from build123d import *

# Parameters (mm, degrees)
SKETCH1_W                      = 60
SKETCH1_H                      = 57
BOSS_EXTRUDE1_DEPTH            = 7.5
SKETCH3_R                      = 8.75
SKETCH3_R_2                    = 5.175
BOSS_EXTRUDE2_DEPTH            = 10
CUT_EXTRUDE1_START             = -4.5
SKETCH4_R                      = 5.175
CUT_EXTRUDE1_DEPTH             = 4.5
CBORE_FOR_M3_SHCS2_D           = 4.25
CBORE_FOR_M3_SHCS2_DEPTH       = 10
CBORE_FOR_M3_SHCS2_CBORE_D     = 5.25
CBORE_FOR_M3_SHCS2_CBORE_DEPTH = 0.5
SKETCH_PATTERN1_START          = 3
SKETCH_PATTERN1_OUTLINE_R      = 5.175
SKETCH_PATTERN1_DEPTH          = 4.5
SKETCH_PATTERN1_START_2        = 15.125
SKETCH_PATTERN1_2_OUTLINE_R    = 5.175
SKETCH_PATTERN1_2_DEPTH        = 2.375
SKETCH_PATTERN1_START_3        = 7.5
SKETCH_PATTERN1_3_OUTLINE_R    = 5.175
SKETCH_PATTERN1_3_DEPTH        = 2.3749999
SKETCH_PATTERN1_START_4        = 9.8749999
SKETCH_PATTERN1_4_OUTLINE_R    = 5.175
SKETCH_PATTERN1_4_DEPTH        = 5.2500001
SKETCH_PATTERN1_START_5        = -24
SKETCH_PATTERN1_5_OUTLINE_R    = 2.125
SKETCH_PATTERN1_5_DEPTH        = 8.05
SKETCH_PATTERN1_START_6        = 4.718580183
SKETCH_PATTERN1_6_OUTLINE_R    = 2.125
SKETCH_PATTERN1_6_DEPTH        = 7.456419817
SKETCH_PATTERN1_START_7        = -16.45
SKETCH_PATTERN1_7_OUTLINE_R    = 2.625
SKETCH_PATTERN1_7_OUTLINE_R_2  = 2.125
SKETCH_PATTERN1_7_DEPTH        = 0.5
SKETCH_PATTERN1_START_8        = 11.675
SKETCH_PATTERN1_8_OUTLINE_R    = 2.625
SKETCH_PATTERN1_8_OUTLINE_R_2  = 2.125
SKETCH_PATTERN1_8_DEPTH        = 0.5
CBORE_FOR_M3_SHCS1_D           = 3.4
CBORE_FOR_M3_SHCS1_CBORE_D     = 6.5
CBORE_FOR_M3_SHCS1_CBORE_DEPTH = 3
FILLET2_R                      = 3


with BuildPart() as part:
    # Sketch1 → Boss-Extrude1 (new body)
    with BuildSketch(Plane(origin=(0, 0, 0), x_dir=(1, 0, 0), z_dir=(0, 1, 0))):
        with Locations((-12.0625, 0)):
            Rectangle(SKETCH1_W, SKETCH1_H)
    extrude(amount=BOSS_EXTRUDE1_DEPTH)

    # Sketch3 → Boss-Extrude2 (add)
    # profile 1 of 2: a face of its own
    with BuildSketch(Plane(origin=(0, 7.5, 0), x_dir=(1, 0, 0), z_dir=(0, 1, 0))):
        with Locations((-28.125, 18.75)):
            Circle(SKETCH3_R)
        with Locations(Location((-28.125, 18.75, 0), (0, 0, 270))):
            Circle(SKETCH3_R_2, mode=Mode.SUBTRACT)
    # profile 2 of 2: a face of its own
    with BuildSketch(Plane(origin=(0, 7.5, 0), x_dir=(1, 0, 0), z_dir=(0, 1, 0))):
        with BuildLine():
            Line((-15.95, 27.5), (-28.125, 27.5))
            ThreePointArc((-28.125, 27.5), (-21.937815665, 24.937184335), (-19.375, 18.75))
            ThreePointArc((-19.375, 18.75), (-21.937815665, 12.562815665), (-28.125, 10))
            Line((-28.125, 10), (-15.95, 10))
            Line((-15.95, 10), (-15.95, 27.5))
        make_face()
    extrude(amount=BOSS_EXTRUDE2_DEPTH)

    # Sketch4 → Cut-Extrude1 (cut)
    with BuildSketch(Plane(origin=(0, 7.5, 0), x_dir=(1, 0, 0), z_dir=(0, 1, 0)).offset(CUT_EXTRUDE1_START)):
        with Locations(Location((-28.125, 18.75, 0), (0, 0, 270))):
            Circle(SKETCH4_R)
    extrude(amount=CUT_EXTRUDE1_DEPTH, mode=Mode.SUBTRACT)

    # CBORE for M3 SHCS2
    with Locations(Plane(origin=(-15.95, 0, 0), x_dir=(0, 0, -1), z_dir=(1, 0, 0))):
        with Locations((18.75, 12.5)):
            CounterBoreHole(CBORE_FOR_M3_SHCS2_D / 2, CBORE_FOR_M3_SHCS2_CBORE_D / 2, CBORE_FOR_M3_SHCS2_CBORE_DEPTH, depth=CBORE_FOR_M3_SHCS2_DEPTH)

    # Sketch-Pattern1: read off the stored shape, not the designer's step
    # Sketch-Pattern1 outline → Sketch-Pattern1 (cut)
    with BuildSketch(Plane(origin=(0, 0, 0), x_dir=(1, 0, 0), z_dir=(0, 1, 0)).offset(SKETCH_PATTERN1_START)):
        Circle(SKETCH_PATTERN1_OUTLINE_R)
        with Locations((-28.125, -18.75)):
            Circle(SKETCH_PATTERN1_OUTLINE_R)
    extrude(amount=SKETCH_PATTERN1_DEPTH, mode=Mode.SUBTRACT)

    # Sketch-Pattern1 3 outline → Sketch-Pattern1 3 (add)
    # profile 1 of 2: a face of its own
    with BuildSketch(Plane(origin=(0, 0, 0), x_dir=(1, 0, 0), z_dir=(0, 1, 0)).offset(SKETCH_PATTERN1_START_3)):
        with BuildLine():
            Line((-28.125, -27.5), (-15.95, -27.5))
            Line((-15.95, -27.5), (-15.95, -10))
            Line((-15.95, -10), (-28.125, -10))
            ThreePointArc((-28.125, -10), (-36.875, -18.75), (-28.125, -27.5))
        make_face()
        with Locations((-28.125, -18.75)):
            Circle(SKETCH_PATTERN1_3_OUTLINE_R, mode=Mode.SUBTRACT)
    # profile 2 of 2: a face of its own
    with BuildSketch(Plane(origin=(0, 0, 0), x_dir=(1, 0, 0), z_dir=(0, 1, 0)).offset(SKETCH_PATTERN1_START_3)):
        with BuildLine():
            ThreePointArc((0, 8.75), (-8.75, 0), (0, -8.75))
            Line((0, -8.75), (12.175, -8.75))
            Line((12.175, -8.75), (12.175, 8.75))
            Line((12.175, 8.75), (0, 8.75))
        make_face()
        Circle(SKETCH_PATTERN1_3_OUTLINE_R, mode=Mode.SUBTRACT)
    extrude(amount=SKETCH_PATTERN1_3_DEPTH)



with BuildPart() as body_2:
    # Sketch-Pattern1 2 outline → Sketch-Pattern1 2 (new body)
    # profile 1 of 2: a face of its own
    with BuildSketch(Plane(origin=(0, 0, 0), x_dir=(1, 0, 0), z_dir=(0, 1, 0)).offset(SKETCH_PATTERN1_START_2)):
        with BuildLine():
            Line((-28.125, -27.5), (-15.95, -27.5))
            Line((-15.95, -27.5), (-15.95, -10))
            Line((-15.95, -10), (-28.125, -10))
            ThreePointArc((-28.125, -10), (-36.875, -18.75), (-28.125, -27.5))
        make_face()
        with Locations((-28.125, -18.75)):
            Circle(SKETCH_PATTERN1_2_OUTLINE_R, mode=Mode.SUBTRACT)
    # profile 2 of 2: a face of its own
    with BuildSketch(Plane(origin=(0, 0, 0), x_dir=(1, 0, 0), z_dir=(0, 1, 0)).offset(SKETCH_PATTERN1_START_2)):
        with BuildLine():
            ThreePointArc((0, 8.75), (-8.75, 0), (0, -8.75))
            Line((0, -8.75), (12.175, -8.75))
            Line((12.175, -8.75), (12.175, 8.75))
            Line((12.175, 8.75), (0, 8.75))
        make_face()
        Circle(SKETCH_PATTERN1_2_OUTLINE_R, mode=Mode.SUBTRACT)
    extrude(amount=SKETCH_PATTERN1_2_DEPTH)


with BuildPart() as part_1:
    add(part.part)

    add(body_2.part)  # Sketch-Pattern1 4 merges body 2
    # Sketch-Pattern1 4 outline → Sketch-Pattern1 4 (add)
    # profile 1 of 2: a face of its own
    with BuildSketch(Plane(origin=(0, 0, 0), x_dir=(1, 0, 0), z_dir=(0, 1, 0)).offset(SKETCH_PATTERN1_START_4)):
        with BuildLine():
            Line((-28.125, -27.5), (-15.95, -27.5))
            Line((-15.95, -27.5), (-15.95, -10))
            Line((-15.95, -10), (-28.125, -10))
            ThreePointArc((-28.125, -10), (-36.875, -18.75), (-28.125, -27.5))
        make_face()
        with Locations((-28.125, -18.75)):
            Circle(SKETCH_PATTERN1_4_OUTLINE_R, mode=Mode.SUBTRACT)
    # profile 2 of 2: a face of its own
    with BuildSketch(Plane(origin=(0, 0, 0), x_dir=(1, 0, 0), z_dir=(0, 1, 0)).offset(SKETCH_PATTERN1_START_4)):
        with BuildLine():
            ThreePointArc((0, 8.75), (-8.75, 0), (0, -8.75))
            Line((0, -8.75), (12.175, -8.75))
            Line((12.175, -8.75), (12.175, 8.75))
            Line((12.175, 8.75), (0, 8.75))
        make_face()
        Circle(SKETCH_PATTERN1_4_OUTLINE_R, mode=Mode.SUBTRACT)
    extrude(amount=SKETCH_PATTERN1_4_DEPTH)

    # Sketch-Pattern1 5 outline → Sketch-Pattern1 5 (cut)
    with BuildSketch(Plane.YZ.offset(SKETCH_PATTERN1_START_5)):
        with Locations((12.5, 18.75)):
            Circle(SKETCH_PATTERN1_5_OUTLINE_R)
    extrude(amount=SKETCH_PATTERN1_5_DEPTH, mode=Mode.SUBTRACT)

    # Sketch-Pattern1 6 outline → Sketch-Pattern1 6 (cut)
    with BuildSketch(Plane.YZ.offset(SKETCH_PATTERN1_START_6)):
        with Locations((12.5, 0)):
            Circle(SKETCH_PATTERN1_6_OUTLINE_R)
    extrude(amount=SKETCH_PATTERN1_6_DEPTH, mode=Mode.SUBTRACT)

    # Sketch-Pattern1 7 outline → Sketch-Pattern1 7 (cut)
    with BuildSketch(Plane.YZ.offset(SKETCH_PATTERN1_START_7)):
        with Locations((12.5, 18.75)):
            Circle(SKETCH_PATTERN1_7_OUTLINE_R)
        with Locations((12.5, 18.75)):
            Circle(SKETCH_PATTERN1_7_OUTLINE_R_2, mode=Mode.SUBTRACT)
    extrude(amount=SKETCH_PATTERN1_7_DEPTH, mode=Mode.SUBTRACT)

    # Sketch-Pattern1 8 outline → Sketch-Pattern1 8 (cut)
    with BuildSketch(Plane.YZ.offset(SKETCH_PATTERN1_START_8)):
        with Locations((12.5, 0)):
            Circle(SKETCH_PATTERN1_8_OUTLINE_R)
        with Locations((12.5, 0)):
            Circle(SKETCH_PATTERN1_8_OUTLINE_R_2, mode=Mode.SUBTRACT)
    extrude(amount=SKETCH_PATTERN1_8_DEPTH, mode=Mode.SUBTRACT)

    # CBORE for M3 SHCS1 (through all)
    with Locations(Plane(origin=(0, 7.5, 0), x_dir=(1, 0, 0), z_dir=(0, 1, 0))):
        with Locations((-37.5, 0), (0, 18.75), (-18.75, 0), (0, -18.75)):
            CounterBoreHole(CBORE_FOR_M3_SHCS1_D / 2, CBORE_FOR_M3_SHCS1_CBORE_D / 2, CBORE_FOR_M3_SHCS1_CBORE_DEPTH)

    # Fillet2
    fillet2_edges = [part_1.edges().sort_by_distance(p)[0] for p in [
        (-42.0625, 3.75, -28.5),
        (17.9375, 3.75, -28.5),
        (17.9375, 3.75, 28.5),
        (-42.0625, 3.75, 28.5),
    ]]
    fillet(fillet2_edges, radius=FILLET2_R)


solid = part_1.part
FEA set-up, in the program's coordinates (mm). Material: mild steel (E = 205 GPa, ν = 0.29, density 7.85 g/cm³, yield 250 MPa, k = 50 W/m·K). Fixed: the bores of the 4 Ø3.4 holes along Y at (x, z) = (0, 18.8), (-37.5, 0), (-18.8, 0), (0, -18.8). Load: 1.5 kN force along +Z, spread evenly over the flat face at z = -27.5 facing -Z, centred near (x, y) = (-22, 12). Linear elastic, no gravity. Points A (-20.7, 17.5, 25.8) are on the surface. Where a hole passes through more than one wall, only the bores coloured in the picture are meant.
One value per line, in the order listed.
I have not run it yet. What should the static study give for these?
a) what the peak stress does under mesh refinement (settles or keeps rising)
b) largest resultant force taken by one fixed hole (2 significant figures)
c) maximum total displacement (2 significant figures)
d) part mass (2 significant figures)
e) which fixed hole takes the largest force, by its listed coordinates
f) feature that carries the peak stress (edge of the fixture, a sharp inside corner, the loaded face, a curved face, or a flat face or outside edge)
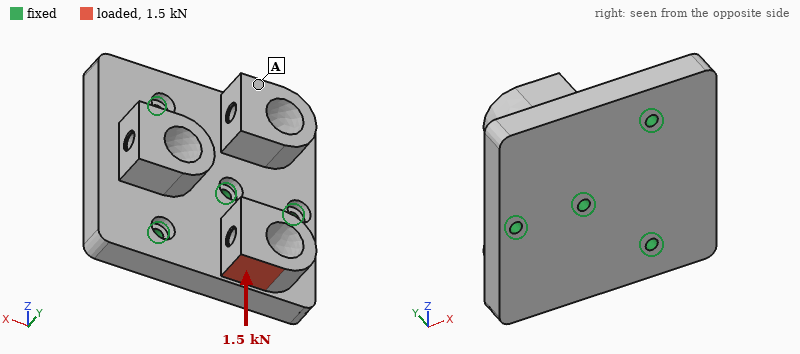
keeps rising
760 N
15 µm
240 g
(-18.8, 0)
edge of the fixture
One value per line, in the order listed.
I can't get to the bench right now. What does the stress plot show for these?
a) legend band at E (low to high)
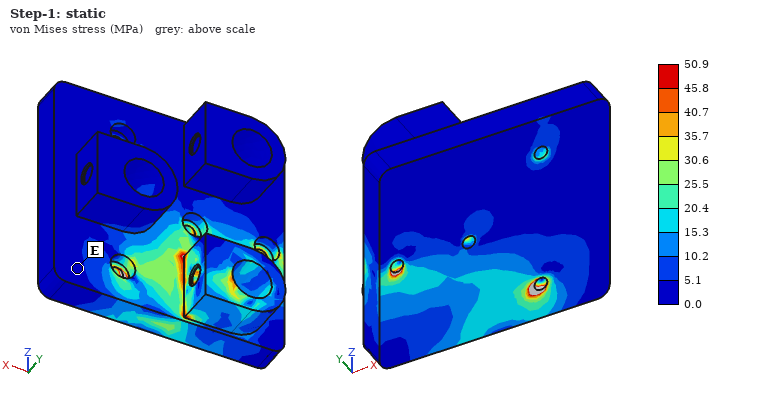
0.0 to 5.1 MPa
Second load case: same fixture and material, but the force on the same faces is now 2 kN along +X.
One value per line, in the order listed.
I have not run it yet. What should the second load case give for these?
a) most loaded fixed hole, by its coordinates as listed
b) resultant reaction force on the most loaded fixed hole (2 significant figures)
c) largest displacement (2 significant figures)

(0, -18.8)
1.4 kN
13 µm
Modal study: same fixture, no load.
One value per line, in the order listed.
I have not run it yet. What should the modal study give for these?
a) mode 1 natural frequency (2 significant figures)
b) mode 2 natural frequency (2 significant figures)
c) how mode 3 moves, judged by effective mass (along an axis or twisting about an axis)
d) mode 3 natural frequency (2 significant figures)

6400 Hz
7200 Hz
along Y
10 kHz
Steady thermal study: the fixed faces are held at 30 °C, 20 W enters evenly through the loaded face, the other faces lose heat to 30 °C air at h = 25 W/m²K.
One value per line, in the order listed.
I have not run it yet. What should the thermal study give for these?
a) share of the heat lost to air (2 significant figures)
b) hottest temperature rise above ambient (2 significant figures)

11 %
54 K
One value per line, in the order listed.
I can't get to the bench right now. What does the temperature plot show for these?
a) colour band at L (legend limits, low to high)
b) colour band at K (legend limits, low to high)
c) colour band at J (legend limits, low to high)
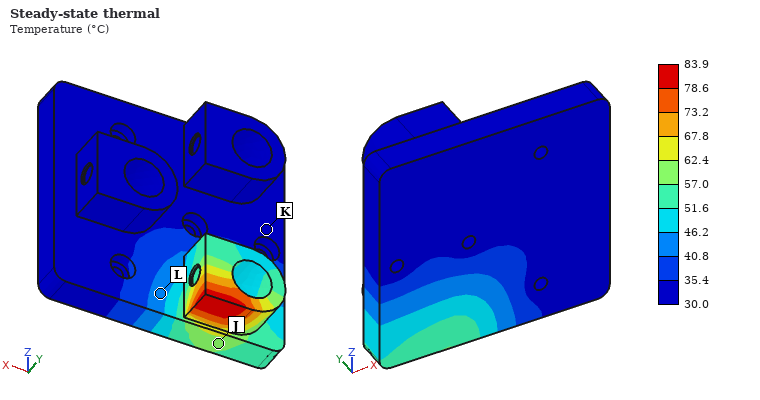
40.8 to 46.2 °C
30.0 to 35.4 °C
57.0 to 62.4 °C
